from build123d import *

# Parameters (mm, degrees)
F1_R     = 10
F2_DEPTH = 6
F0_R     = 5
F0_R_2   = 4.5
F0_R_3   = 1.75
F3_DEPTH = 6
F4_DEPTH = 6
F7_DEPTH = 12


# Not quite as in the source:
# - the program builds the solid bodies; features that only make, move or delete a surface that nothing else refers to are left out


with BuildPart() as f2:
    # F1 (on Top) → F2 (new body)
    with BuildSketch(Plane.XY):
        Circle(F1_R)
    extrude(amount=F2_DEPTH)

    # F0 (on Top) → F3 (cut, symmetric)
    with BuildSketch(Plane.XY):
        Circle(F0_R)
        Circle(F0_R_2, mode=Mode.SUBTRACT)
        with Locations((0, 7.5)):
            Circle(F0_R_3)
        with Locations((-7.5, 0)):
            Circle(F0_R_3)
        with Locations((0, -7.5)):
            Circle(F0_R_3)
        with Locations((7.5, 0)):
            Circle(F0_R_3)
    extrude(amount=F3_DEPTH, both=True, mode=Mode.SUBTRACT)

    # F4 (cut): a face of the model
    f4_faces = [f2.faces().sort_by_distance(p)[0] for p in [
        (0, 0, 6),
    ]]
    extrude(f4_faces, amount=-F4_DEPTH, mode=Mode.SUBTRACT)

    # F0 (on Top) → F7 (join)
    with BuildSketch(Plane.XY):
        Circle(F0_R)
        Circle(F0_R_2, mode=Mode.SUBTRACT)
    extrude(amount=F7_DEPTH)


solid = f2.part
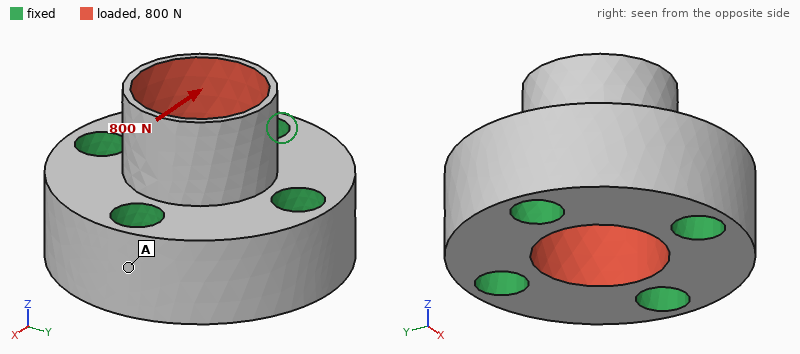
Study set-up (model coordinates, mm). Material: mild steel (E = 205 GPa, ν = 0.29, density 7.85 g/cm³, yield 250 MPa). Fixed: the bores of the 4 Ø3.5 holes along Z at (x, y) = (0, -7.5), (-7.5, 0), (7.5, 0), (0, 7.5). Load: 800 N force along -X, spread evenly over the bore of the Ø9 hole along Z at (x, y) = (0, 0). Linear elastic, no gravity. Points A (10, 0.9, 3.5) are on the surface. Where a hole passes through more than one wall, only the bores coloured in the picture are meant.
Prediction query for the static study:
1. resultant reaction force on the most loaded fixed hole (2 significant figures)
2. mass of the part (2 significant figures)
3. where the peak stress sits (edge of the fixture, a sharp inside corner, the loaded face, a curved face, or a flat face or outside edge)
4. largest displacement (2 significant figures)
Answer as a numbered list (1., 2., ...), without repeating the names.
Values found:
1. 240 N
2. 11 g
3. the loaded face
4. 3.4 µm
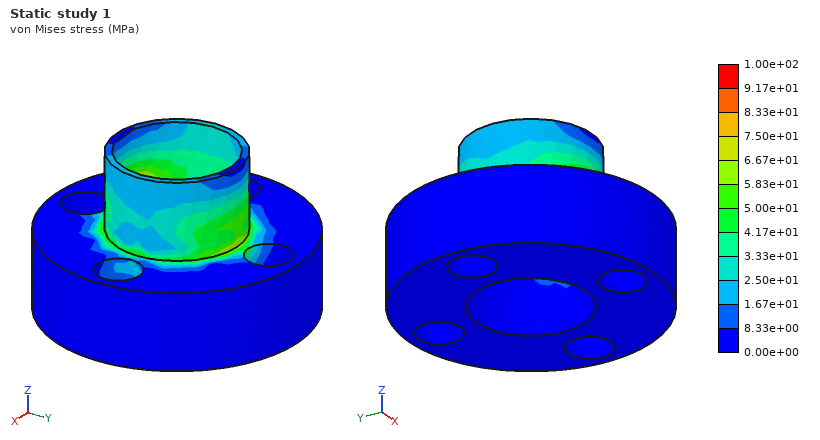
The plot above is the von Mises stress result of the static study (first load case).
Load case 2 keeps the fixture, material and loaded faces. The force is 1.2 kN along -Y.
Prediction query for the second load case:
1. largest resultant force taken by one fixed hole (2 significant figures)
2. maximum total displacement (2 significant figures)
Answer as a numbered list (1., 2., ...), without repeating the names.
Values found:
1. 360 N
2. 5.0 µm
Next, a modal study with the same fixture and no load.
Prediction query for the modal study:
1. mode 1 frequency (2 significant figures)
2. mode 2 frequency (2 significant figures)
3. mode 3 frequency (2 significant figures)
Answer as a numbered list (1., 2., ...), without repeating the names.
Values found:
1. 49 kHz
2. 50 kHz
3. 57 kHz
